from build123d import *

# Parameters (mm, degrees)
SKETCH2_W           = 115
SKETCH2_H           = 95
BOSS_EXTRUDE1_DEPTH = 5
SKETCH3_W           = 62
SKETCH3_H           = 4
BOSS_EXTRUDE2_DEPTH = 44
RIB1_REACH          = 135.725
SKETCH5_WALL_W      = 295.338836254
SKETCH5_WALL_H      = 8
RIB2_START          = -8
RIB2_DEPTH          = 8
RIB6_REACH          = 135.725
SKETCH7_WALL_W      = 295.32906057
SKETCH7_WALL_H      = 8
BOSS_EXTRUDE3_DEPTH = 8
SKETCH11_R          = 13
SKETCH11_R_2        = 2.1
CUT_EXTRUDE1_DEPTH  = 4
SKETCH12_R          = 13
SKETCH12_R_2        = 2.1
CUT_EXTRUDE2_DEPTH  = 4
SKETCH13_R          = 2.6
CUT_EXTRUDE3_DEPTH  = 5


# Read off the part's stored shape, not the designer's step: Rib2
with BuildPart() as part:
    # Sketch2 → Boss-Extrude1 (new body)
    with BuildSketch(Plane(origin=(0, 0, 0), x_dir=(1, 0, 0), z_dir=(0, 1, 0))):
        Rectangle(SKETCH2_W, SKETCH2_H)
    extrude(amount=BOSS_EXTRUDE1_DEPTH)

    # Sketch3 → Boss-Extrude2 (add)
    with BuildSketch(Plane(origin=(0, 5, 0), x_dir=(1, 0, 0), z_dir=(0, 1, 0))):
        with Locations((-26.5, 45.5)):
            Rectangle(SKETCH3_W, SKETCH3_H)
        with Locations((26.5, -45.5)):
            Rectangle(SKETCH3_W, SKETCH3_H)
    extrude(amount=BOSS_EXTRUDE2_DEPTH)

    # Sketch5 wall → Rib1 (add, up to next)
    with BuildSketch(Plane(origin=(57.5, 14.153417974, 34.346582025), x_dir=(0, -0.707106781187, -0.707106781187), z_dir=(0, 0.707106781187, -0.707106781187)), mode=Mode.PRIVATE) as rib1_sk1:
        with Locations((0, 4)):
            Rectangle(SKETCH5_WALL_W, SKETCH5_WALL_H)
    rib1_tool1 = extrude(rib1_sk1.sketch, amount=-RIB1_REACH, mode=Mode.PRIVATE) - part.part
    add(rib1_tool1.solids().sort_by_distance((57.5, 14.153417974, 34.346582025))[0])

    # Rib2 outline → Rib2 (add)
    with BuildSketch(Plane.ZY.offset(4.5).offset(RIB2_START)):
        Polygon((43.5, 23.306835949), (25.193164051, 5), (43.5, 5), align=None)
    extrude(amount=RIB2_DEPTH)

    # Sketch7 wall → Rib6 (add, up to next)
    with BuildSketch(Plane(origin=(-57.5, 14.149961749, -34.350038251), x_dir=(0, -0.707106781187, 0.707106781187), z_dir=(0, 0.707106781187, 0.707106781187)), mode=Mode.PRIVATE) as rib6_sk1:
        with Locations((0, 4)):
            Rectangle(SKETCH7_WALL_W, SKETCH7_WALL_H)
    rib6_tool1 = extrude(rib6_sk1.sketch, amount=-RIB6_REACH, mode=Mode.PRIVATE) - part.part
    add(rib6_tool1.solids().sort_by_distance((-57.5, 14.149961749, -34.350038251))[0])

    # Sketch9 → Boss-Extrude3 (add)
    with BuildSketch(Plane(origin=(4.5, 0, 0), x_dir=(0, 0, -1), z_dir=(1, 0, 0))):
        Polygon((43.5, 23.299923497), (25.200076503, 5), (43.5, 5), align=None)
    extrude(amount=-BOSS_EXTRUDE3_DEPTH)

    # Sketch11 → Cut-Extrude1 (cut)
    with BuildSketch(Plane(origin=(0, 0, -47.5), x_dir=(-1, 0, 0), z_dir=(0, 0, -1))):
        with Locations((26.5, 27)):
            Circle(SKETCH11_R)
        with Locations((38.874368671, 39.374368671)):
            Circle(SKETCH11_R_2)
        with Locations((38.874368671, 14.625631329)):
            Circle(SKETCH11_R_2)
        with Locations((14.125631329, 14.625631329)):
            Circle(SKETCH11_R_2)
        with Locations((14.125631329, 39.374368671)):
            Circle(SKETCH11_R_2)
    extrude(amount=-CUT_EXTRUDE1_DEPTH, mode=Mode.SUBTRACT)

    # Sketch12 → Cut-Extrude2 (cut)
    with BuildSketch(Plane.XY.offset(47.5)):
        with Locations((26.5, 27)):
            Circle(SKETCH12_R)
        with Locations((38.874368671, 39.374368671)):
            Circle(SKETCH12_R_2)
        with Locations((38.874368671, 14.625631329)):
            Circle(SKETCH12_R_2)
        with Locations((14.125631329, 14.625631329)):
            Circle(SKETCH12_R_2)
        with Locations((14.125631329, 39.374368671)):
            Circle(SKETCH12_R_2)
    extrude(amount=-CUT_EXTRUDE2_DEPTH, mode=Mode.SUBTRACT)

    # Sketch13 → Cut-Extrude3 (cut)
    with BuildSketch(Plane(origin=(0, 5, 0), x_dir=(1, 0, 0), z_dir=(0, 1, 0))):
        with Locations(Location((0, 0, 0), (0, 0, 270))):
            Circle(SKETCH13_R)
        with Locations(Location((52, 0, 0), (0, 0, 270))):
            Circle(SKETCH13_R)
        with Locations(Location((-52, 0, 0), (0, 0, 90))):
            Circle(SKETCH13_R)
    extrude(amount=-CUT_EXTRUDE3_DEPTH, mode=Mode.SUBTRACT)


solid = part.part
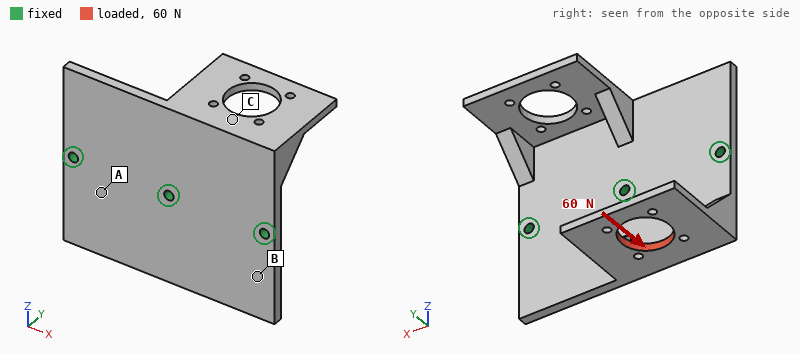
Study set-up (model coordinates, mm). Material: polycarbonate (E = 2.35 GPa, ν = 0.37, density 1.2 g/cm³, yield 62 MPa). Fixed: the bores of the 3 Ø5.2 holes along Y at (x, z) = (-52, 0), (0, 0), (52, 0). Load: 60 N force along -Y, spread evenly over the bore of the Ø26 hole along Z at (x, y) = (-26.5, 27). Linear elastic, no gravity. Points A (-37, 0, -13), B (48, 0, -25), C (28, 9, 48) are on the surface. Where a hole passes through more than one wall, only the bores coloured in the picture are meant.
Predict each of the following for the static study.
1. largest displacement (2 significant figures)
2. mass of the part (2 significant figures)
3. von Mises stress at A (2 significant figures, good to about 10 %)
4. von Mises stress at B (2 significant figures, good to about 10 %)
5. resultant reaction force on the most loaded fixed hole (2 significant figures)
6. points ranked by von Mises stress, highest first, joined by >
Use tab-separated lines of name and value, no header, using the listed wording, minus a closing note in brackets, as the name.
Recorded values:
largest displacement	1.8 mm
mass of the part	92 g
von Mises stress at A	4.4 MPa
von Mises stress at B	1.8 MPa
resultant reaction force on the most loaded fixed hole	31 N
points ranked by von Mises stress, highest first, joined by >	A > B > C
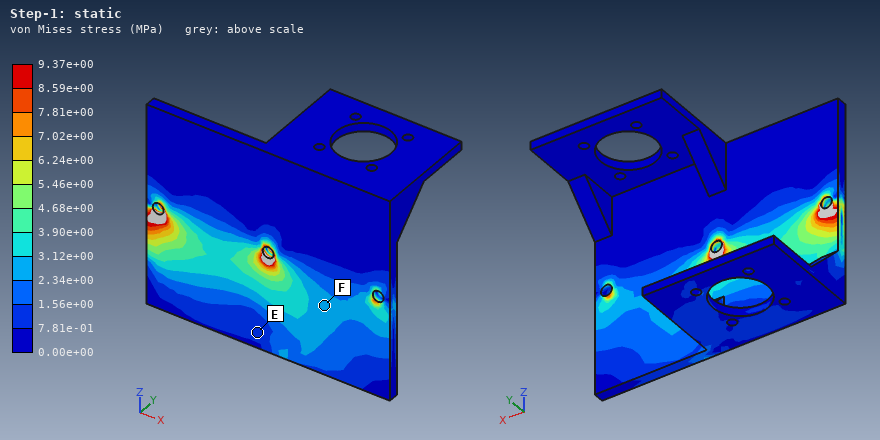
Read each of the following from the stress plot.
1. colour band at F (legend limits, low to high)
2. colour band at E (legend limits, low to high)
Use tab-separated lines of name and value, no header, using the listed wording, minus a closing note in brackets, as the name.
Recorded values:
colour band at F	2.34e+00 to 3.12e+00 MPa
colour band at E	7.81e-01 to 1.56e+00 MPa
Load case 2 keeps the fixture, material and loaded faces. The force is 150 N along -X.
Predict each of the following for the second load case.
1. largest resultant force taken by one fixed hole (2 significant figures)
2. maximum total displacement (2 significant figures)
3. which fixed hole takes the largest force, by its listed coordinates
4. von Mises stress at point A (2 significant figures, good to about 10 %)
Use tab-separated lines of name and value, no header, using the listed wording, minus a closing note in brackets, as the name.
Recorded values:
largest resultant force taken by one fixed hole	100 N
maximum total displacement	1.5 mm
which fixed hole takes the largest force, by its listed coordinates	(-52, 0)
von Mises stress at point A	3.5 MPa
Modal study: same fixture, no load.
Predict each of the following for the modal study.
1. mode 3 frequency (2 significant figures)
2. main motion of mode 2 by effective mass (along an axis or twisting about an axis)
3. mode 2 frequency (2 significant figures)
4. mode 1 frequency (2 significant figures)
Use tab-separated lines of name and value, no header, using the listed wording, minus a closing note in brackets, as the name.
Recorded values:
mode 3 frequency	450 Hz
main motion of mode 2 by effective mass	along Y
mode 2 frequency	270 Hz
mode 1 frequency	220 Hz
